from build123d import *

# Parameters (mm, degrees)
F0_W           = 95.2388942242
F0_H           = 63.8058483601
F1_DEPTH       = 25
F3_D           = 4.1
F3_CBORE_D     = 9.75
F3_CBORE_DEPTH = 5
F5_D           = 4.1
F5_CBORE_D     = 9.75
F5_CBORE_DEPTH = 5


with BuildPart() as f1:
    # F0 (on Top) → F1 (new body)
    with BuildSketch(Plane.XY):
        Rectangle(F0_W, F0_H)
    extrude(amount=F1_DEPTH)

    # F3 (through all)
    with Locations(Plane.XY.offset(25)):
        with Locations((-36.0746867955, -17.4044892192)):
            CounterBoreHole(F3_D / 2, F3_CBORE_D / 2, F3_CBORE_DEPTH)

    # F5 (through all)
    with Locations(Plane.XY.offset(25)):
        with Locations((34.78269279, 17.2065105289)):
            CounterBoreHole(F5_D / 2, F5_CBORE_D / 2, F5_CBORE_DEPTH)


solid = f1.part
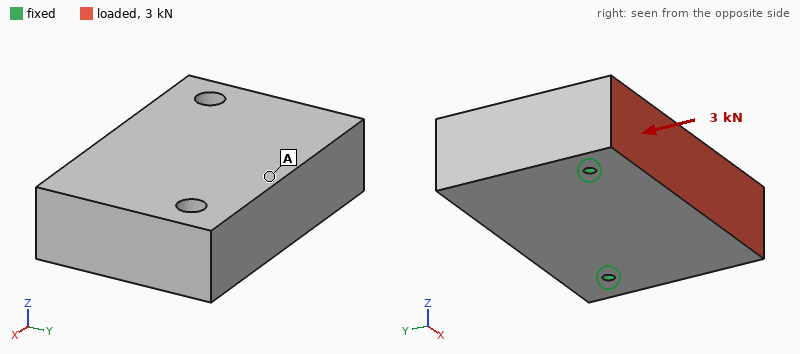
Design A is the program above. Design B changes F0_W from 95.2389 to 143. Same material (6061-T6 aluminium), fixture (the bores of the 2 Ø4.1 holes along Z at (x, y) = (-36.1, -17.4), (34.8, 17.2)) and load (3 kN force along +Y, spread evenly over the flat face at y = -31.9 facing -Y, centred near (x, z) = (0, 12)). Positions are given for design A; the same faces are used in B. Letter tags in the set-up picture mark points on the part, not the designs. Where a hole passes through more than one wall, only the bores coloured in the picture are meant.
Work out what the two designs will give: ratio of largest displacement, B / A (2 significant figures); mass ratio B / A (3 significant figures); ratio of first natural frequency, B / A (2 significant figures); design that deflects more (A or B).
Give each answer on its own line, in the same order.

1.2
1.51
0.73
B
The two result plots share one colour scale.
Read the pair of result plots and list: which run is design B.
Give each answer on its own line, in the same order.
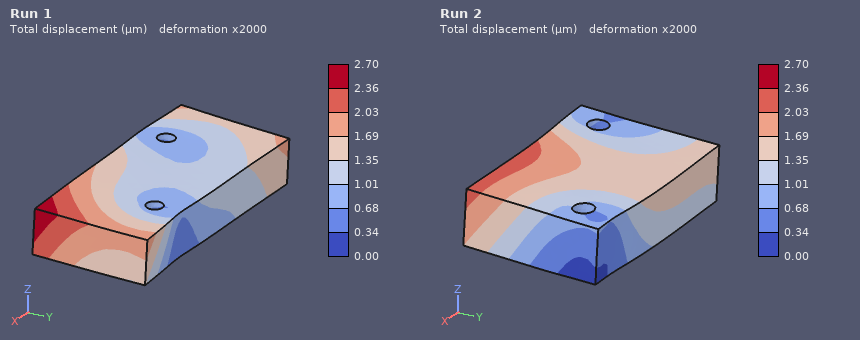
Run 1
